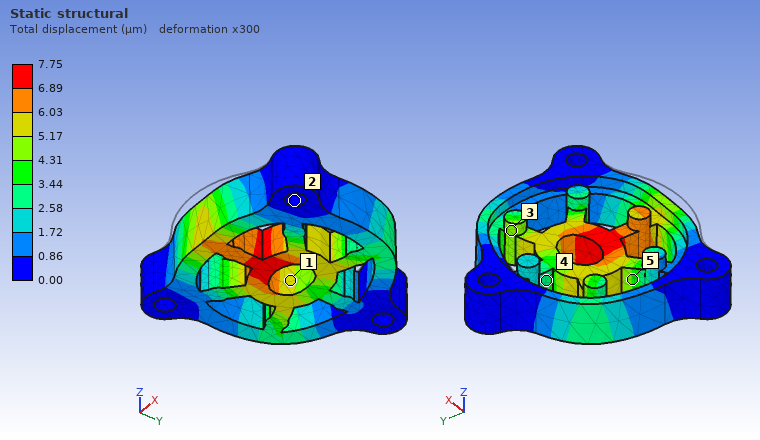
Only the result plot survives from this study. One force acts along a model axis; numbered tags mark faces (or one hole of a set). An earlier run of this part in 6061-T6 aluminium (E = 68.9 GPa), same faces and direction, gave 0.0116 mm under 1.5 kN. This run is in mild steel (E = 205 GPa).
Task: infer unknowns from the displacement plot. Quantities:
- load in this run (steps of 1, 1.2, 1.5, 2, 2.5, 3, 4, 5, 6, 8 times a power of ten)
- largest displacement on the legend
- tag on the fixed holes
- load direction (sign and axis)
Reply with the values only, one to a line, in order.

3 kN
7.75 µm
2
+Y
